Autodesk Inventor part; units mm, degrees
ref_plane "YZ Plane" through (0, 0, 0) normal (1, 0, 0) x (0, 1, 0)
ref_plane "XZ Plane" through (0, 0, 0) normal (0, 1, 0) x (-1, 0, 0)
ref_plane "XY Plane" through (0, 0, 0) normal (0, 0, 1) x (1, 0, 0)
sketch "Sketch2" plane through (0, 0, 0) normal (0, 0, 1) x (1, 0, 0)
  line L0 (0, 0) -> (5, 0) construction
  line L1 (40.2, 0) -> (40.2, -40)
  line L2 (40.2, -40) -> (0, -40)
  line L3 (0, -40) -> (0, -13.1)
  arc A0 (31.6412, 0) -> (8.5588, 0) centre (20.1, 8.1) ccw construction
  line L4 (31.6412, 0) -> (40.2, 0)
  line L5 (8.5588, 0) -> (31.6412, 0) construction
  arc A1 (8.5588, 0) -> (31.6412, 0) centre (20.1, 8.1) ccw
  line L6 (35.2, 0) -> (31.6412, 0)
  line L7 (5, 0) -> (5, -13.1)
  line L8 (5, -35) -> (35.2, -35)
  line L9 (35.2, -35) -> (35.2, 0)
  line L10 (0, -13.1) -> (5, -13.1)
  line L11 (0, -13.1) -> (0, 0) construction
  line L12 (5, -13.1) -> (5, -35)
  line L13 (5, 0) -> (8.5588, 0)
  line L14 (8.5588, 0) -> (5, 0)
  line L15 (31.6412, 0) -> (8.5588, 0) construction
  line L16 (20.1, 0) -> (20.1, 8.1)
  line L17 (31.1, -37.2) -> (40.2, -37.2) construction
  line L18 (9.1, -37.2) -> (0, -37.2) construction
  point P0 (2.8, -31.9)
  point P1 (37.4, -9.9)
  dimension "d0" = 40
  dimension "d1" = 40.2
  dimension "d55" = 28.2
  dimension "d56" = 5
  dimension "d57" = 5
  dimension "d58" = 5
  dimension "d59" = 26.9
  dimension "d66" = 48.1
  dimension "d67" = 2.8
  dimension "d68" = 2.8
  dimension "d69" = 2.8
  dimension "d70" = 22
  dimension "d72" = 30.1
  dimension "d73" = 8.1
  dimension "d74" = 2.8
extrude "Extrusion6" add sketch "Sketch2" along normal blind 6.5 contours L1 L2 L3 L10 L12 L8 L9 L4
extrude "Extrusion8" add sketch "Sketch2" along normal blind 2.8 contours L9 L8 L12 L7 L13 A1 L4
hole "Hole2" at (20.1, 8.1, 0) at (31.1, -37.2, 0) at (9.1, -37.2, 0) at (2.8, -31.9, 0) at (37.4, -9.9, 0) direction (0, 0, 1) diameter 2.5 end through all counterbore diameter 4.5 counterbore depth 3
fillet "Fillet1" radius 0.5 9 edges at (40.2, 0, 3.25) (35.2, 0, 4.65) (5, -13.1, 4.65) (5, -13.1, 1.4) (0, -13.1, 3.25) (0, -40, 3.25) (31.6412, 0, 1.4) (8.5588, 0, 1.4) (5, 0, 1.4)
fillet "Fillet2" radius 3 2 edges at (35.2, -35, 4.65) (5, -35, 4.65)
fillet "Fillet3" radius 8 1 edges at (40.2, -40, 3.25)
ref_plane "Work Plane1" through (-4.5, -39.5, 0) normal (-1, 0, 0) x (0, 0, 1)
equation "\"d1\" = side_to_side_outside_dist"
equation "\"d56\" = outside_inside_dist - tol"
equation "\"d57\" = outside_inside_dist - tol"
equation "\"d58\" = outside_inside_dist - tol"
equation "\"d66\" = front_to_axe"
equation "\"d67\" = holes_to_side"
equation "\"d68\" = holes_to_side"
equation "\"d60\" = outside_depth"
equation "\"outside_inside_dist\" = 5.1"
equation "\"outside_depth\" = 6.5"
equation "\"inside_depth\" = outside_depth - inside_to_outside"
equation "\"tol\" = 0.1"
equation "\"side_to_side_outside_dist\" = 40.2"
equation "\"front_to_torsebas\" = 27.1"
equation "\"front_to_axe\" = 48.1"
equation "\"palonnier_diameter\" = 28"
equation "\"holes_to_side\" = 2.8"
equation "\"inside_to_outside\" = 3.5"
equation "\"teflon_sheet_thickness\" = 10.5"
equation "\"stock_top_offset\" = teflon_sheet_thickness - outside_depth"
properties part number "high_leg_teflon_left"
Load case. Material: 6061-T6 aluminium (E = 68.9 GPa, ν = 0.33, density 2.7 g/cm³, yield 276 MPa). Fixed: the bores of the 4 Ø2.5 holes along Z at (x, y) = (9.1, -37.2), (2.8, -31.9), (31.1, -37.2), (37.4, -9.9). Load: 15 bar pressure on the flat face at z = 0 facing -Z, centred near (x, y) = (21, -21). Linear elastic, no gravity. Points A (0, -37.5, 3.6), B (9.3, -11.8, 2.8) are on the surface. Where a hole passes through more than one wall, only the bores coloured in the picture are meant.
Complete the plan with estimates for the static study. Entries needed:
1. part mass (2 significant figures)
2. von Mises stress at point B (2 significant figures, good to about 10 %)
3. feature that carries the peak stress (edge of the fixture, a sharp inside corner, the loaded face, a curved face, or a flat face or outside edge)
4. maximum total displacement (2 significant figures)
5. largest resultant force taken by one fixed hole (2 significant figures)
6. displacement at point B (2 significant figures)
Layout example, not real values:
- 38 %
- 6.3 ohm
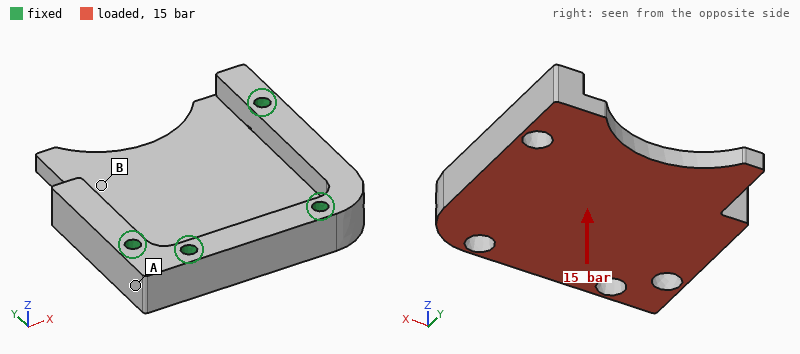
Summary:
- 15 g
- 57 MPa
- a curved face
- 0.28 mm
- 1.2 kN
- 0.14 mm
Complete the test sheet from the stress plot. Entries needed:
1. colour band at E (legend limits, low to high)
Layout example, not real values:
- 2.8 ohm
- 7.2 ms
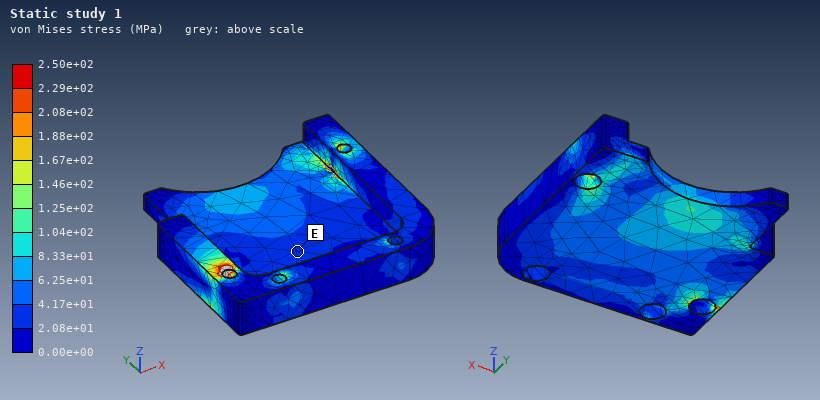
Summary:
- 2.08e+01 to 4.17e+01 MPa
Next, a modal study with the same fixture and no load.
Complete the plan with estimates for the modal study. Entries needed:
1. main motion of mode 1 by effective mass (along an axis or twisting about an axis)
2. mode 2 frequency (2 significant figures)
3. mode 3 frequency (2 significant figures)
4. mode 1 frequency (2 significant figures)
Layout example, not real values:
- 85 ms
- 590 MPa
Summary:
- along Z
- 14 kHz
- 15 kHz
- 6100 Hz
